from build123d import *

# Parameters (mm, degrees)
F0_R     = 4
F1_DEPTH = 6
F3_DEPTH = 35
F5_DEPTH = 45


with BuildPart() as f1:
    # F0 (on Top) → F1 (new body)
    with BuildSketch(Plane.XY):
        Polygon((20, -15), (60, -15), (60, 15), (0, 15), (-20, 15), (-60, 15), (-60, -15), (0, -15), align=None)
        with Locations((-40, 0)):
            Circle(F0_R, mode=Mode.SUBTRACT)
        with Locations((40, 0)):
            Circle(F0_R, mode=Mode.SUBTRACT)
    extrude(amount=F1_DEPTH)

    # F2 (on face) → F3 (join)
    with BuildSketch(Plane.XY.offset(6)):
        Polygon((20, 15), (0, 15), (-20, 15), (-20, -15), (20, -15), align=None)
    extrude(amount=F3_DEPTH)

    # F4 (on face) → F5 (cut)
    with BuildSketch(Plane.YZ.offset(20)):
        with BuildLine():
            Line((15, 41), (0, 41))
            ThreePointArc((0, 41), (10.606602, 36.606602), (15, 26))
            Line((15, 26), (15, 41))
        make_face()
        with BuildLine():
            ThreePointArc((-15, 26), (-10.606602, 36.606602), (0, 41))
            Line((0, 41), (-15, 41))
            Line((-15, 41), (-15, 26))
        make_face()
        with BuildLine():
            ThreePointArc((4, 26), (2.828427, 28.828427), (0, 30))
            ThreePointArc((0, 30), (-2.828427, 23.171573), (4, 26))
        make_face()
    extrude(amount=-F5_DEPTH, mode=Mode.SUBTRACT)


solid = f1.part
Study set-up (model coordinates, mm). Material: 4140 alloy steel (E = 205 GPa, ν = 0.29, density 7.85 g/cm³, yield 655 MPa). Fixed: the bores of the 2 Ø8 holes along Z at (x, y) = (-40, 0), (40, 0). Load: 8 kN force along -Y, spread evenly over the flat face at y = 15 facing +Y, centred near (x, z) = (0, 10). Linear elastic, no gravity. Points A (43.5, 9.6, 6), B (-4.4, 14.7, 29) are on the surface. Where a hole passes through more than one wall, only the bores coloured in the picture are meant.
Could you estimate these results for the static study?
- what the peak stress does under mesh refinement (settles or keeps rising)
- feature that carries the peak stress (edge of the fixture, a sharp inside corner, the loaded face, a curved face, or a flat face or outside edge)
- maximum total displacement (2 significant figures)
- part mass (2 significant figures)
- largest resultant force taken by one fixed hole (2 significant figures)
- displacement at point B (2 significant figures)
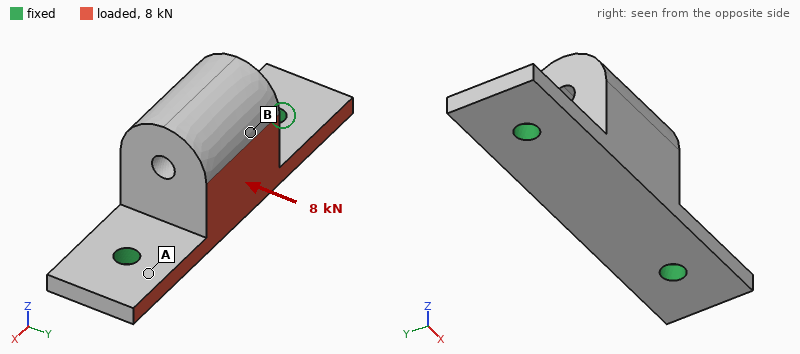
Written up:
keeps rising
edge of the fixture
0.12 mm
450 g
4.0 kN
0.093 mm
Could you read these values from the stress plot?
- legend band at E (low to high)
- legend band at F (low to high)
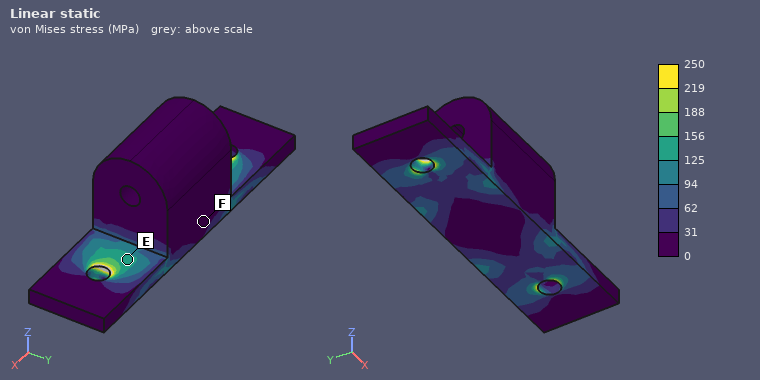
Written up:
125 to 156 MPa
0 to 31 MPa
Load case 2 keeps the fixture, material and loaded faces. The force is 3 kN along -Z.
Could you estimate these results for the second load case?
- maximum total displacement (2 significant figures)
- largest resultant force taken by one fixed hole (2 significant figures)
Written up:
67 µm
1.6 kN
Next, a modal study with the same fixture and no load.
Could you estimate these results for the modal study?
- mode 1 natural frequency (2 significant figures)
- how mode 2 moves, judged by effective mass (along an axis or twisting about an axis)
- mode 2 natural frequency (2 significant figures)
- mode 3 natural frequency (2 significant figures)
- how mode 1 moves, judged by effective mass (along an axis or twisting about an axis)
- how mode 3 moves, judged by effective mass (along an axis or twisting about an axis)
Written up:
1800 Hz
along Z
3800 Hz
4800 Hz
along Y
along X
